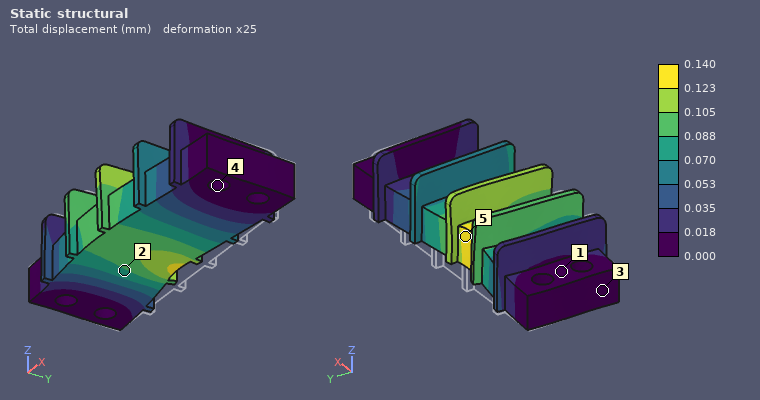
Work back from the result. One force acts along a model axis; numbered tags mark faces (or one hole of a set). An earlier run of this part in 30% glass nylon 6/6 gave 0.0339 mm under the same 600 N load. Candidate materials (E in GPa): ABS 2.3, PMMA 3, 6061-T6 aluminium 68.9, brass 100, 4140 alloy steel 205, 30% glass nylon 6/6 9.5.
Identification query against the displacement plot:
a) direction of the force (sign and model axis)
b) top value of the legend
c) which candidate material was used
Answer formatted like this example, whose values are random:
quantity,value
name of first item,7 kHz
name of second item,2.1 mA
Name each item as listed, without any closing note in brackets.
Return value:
quantity,value
direction of the force,-Y
top value of the legend,0.140 mm
which candidate material was used,ABS
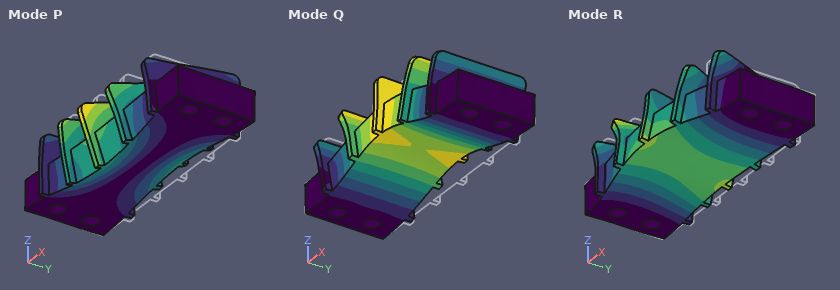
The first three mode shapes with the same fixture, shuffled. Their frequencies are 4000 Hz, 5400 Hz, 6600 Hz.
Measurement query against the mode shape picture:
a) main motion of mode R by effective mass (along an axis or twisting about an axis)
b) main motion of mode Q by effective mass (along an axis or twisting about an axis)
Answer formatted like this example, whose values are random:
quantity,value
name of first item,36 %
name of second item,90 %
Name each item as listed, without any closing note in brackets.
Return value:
quantity,value
main motion of mode R by effective mass,along Y
main motion of mode Q by effective mass,along Z
